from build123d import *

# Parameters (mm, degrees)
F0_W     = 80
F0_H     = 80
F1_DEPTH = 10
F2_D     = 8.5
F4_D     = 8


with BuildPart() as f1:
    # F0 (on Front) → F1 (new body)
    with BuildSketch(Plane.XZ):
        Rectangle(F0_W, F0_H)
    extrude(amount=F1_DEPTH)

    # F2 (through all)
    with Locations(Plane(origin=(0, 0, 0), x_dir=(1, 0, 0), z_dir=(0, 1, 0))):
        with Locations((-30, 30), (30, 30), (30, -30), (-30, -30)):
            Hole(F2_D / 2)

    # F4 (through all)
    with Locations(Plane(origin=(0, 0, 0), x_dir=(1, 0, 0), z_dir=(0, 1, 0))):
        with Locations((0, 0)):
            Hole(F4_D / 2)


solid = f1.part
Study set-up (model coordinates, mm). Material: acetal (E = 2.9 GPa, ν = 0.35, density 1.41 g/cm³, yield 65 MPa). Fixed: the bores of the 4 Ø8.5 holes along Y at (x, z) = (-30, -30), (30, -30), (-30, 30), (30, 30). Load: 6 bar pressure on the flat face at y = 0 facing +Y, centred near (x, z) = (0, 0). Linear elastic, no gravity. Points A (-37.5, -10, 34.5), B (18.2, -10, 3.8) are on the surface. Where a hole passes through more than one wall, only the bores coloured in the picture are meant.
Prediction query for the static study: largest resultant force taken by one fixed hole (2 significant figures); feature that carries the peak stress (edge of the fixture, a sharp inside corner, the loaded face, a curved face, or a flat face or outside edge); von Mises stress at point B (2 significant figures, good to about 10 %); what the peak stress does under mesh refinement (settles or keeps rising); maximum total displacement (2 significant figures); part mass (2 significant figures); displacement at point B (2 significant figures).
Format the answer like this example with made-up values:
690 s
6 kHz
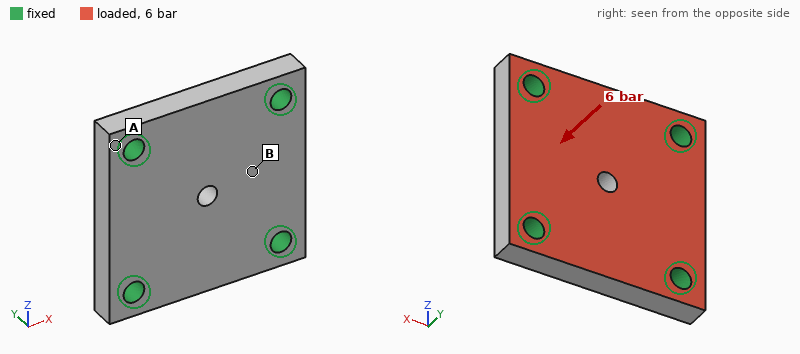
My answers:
920 N
edge of the fixture
5.2 MPa
keeps rising
0.22 mm
86 g
0.16 mm
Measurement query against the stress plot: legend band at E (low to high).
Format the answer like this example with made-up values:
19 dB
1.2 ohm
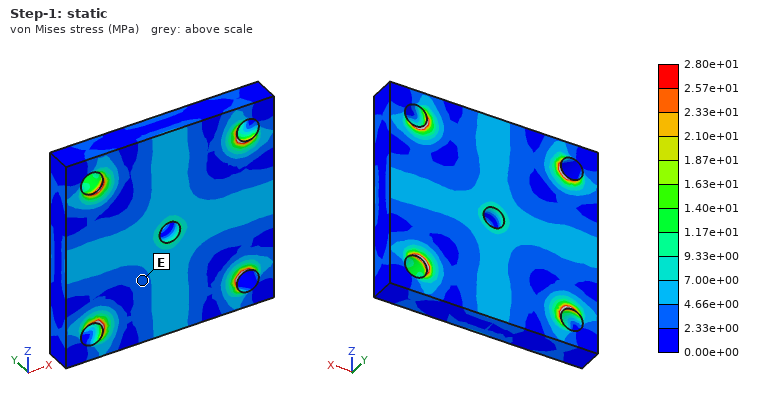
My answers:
2.33e+00 to 4.66e+00 MPa
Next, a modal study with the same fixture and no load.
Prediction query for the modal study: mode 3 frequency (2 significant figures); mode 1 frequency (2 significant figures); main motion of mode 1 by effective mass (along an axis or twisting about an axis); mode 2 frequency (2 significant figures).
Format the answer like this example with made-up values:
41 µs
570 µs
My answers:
4200 Hz
2800 Hz
along Y
4200 Hz
